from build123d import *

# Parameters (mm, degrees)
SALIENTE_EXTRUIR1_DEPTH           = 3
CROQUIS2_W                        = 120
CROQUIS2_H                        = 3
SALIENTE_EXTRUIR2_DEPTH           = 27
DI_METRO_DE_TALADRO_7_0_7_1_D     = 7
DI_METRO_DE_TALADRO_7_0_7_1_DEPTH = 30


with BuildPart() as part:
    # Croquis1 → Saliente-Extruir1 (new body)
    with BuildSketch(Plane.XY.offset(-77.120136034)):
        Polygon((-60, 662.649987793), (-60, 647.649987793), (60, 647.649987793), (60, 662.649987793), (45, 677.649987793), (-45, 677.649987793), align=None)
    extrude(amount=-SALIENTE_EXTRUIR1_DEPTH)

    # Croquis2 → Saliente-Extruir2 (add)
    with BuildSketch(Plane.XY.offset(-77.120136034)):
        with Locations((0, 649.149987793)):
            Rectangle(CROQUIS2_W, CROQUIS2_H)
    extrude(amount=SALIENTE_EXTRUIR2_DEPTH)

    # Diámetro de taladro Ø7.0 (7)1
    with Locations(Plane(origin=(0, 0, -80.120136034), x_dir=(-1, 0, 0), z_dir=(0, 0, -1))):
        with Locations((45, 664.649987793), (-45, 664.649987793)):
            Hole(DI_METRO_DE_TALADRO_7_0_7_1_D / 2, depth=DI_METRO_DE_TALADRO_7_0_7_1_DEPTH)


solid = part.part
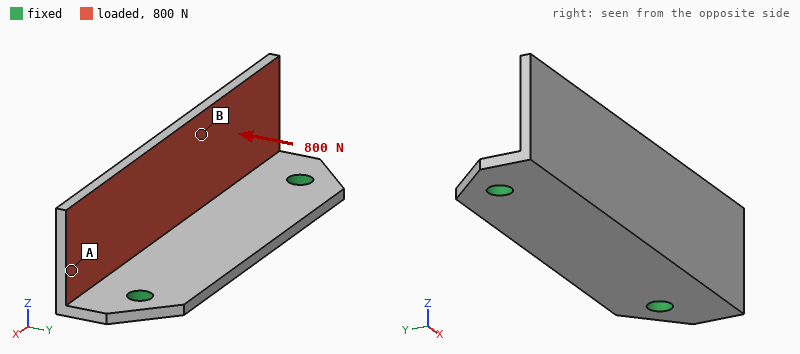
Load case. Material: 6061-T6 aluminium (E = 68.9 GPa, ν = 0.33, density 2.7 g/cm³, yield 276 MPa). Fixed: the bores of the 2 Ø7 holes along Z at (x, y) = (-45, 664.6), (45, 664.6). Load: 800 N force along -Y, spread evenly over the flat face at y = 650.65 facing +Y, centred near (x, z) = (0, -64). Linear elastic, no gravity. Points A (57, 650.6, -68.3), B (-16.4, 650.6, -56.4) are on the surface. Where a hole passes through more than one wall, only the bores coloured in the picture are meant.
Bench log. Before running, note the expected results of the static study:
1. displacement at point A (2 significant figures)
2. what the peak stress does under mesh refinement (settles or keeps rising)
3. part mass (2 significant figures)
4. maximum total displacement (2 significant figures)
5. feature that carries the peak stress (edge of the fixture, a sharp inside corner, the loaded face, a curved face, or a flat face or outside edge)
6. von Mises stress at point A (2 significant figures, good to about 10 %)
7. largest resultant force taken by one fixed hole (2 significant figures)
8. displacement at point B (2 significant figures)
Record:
0.15 mm
keeps rising
53 g
0.51 mm
edge of the fixture
29 MPa
400 N
0.38 mm
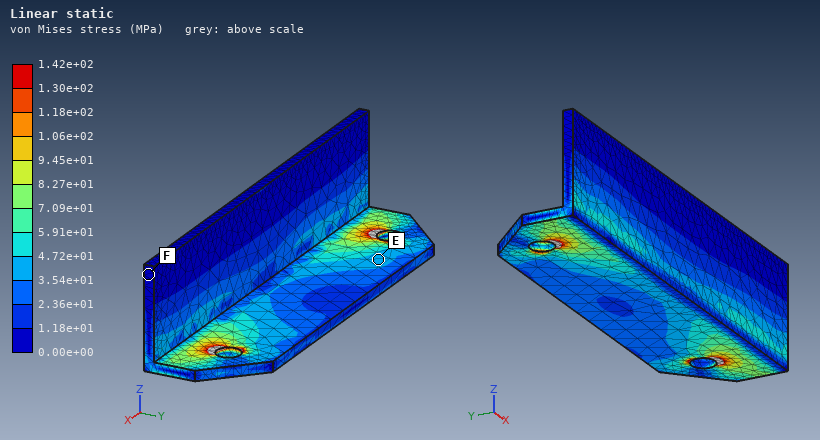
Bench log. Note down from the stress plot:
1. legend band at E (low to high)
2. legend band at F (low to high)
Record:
3.54e+01 to 4.72e+01 MPa
0.00e+00 to 1.18e+01 MPa
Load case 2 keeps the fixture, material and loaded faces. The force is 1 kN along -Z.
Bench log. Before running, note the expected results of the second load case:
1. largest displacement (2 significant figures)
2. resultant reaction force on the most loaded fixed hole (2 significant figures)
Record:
0.21 mm
510 N
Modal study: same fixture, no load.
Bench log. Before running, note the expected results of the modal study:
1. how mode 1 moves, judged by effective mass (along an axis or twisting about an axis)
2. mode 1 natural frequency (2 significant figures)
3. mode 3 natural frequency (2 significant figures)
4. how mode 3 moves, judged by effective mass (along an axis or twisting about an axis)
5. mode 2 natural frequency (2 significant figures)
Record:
along Y
1400 Hz
2900 Hz
along Z
2200 Hz
